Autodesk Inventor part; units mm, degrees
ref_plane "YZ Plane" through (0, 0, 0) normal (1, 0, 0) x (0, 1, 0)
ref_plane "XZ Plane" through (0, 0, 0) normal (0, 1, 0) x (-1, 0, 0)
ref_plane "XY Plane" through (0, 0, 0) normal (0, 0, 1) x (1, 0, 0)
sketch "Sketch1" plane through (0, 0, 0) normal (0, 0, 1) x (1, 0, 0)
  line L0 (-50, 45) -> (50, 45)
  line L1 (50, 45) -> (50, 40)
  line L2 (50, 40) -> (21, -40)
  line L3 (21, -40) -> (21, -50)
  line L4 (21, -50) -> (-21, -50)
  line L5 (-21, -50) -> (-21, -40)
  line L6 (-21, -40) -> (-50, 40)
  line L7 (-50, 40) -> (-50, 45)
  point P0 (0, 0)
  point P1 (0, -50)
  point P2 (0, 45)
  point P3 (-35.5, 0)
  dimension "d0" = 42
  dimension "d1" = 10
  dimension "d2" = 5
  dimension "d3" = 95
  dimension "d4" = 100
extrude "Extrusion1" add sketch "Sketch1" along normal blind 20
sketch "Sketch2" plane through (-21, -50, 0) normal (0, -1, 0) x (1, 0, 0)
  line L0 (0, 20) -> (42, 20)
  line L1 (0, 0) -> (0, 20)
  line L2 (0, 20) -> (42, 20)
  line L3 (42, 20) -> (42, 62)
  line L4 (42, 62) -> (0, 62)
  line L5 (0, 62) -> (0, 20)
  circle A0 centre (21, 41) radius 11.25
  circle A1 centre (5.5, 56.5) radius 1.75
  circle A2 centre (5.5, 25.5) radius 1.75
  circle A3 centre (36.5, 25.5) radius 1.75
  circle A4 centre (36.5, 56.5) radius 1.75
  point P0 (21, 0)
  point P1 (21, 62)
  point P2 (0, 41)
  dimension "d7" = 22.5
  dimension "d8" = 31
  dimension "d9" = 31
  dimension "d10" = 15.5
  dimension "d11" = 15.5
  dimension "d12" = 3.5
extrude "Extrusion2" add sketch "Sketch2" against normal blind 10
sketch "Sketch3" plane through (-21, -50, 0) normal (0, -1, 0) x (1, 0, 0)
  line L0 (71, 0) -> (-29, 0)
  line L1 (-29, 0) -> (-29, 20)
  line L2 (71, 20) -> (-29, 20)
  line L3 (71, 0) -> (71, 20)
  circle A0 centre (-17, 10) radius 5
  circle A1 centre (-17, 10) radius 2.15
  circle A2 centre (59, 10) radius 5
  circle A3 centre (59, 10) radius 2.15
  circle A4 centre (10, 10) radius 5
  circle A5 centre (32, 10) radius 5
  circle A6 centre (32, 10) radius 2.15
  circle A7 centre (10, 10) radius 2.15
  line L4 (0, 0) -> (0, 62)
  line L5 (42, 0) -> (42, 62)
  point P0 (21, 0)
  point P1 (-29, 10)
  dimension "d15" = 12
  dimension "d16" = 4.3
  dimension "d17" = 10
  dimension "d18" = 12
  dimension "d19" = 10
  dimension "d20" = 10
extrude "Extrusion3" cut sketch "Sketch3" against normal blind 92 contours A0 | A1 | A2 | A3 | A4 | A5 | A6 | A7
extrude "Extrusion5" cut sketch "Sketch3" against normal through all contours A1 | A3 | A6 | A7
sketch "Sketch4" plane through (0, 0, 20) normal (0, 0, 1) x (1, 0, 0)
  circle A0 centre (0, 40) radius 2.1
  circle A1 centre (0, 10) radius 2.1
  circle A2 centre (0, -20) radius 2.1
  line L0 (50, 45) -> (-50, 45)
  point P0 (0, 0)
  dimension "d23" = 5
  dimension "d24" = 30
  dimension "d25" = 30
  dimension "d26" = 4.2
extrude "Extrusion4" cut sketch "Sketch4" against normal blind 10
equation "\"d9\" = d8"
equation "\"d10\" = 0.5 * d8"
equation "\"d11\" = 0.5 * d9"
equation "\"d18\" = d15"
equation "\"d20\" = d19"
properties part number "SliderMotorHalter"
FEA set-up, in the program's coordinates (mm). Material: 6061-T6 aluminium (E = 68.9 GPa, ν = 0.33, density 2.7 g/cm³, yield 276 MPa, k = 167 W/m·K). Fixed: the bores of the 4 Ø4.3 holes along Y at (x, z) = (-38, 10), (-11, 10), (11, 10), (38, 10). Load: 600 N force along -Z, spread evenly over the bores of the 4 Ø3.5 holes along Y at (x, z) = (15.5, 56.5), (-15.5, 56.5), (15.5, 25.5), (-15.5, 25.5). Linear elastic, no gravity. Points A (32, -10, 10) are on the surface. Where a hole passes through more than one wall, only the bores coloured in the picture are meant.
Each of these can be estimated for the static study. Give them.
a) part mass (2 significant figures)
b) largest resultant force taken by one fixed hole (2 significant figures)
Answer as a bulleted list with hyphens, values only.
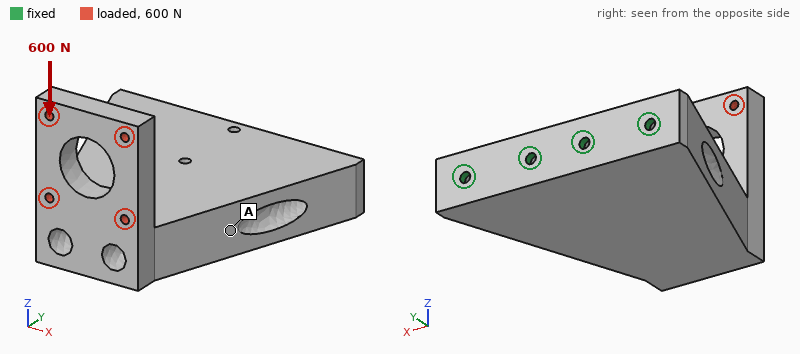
- 340 g
- 280 N
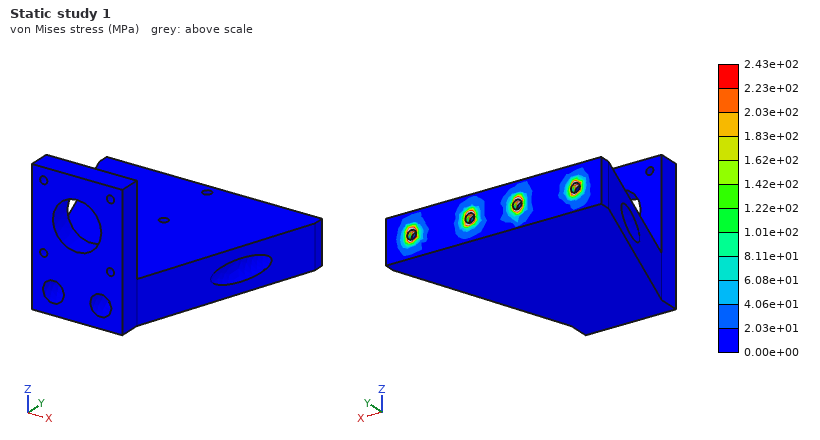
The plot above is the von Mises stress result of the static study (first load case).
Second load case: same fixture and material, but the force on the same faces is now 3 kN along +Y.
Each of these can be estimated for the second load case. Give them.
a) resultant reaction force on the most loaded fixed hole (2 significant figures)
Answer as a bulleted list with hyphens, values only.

- 820 N
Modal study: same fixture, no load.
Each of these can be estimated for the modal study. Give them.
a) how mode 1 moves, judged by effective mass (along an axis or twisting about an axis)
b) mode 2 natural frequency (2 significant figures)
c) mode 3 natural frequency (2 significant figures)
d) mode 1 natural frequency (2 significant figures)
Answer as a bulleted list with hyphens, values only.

- along Z
- 2900 Hz
- 2900 Hz
- 510 Hz
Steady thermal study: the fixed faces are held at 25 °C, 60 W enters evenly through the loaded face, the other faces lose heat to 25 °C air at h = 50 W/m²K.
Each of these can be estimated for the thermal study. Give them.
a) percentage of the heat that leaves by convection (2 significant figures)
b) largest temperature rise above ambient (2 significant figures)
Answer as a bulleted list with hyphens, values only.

- 40 %
- 54 K
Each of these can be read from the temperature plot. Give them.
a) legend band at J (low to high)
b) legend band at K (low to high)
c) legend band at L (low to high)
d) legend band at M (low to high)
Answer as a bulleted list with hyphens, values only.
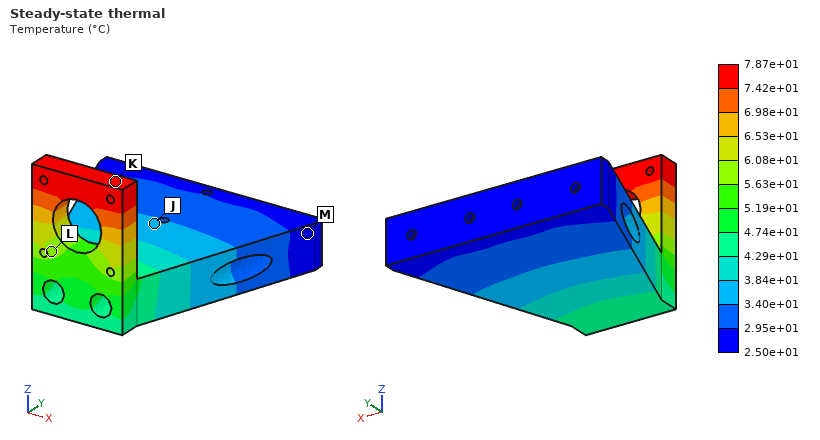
- 3.40e+01 to 3.84e+01 °C
- 7.42e+01 to 7.87e+01 °C
- 5.63e+01 to 6.08e+01 °C
- 2.50e+01 to 2.95e+01 °C
